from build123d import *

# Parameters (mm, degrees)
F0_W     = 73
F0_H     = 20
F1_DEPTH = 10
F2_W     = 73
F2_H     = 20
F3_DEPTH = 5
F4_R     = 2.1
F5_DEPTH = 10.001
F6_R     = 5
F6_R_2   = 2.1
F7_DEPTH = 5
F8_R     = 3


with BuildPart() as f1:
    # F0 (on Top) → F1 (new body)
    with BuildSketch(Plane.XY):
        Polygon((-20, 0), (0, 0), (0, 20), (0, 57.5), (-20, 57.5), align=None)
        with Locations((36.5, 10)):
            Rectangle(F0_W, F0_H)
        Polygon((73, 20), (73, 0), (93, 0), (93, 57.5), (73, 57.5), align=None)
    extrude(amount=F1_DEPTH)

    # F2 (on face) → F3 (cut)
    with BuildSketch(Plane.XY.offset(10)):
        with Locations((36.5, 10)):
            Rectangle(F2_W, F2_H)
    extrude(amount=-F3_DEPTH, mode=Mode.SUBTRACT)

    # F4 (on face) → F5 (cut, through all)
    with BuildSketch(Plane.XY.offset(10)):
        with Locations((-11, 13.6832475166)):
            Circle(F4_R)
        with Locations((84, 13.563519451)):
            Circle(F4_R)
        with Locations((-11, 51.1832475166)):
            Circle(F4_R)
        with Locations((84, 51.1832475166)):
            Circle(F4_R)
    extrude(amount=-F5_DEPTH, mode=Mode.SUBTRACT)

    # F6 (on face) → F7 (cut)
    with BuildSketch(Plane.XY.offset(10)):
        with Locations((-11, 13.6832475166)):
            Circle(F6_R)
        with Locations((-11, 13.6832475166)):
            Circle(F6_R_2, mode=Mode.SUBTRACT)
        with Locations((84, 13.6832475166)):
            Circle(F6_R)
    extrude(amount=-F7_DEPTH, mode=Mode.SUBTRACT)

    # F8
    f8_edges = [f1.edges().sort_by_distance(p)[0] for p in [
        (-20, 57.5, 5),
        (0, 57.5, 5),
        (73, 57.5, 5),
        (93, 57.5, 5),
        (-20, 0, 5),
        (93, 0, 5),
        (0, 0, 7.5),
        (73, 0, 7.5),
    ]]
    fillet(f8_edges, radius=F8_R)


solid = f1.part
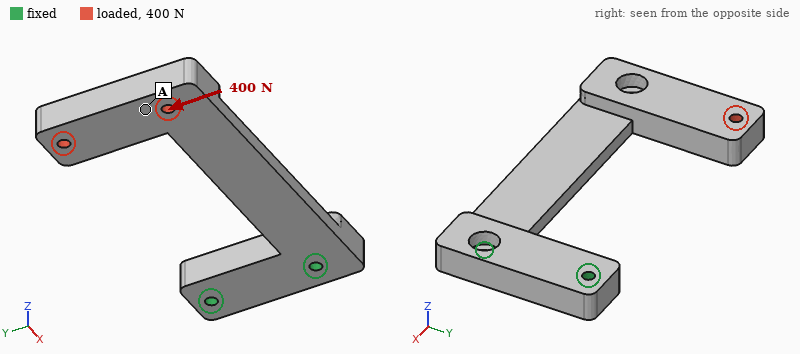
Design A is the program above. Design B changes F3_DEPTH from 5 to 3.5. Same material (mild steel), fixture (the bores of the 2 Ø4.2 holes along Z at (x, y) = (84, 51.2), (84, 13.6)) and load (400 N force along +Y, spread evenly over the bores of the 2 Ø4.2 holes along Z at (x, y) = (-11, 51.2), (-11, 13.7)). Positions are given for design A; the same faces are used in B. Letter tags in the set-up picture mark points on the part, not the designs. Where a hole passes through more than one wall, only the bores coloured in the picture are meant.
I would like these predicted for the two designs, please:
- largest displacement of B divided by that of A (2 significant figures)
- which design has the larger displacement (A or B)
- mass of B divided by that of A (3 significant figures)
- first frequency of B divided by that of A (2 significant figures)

0.78
A
1.08
1.4
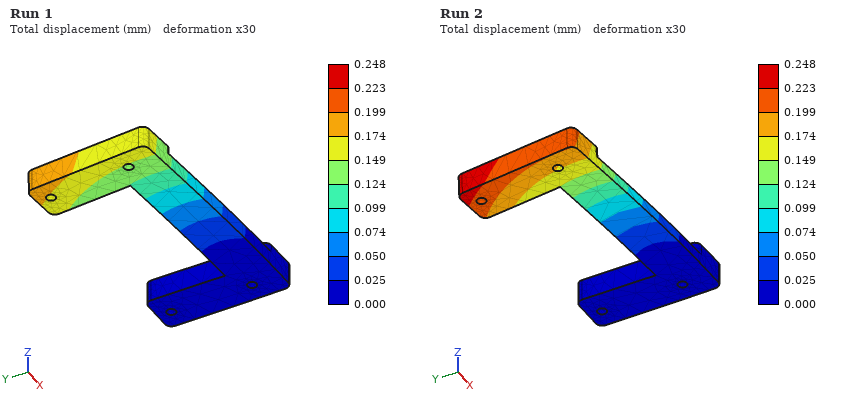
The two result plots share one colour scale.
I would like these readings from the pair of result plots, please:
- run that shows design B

Run 1
